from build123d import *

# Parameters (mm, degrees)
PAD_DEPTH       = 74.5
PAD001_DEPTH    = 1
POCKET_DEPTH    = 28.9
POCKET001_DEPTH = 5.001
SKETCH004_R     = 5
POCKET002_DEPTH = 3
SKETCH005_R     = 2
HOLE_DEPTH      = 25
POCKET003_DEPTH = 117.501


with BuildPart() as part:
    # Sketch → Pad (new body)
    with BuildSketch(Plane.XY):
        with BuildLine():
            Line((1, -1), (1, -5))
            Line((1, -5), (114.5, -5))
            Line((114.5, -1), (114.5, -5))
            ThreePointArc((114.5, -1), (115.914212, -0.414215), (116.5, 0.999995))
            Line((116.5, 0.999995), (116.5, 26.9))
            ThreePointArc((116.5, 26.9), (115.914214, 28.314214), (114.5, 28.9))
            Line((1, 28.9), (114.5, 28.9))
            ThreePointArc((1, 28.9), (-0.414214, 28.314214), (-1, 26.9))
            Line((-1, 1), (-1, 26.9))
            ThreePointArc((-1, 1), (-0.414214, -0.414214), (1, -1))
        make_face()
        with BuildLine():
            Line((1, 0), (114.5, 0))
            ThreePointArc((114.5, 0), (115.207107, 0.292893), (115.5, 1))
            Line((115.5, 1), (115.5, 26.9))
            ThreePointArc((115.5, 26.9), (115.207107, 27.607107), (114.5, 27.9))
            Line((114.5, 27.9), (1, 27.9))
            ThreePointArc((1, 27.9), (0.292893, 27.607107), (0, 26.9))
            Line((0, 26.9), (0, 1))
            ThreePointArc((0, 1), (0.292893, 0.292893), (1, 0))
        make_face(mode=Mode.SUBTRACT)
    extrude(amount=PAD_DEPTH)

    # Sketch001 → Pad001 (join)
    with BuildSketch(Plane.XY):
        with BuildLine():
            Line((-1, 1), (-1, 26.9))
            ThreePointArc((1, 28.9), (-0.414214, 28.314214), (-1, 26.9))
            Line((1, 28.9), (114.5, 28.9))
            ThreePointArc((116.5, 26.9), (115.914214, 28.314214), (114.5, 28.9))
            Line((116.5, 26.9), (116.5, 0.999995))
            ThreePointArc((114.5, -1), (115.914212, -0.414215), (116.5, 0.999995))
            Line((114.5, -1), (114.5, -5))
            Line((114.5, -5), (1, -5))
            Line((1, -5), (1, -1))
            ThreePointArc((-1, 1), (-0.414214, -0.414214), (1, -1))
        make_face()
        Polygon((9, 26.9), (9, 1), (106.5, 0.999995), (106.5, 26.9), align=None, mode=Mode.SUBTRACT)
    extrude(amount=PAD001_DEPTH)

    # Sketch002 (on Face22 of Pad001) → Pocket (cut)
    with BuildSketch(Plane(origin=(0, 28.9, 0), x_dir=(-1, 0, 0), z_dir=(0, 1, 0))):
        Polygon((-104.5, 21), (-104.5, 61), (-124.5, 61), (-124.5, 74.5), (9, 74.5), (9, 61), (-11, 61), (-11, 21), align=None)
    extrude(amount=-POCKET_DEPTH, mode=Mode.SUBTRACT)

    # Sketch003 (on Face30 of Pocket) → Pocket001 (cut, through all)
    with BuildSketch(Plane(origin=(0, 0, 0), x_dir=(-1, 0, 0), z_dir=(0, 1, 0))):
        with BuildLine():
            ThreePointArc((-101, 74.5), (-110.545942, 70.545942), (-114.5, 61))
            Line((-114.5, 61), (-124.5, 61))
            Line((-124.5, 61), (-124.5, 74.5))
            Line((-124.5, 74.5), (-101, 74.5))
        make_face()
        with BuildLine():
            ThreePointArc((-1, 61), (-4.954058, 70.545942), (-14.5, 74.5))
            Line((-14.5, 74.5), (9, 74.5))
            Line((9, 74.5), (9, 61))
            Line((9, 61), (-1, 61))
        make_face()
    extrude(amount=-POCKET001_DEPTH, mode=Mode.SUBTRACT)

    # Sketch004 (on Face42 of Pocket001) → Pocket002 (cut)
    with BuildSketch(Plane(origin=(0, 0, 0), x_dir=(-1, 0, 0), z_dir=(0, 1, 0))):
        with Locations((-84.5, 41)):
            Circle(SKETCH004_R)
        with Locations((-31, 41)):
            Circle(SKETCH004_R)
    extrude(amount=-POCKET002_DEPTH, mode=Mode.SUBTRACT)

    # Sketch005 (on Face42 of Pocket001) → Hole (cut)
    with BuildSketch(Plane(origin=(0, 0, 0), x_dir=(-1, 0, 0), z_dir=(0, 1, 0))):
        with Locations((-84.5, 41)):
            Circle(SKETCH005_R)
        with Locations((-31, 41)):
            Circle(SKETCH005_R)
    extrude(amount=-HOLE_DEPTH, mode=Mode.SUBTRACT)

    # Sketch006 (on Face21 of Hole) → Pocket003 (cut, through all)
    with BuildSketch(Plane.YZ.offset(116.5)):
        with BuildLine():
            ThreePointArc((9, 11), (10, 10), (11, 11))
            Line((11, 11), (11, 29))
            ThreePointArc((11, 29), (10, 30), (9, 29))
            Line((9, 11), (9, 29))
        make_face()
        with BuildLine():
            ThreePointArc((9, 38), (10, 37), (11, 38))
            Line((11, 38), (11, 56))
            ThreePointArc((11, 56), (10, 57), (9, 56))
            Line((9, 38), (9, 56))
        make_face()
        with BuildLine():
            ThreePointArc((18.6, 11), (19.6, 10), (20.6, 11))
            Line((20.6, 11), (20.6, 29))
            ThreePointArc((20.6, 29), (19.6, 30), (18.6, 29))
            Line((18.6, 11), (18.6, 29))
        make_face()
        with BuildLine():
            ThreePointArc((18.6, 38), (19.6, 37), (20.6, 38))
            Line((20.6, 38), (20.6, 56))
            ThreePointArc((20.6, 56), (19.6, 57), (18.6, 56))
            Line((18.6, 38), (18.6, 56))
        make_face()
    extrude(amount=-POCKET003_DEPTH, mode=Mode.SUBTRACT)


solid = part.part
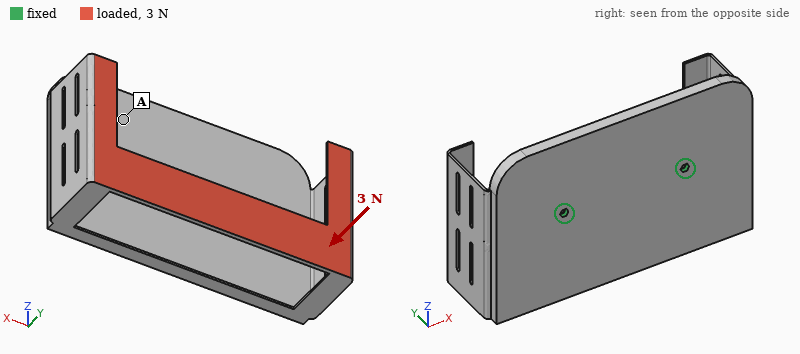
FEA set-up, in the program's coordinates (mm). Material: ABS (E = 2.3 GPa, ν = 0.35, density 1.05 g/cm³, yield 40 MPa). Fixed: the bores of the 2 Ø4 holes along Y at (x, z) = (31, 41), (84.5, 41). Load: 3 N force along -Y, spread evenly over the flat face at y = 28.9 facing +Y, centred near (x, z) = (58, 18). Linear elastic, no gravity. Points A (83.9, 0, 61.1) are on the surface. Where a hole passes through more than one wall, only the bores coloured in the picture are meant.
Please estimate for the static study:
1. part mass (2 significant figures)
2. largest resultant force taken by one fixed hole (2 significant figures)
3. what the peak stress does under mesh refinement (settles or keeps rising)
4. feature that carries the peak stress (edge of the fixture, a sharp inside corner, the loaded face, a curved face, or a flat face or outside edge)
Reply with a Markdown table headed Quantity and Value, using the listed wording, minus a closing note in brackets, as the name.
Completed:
| Quantity | Value |
|---|---|
| part mass | 51 g |
| largest resultant force taken by one fixed hole | 4.2 N |
| what the peak stress does under mesh refinement | keeps rising |
| feature that carries the peak stress | a sharp inside corner |
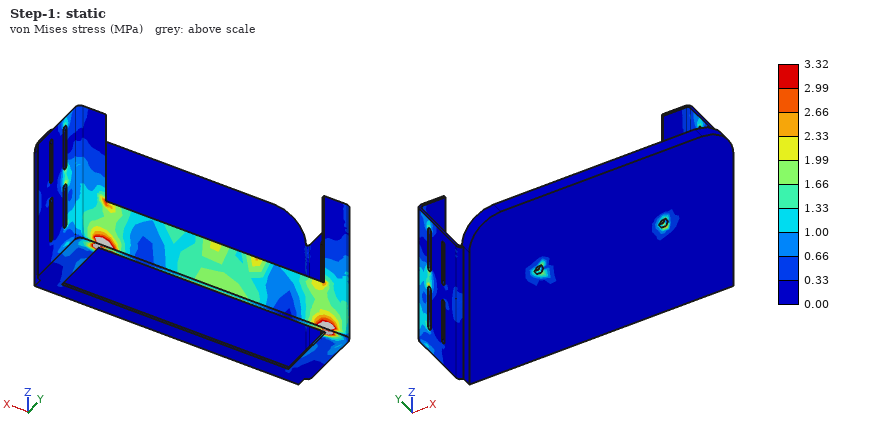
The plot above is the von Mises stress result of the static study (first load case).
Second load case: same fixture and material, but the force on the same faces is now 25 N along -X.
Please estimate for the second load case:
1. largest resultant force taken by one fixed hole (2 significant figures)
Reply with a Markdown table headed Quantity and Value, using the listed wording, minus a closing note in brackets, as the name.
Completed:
| Quantity | Value |
|---|---|
| largest resultant force taken by one fixed hole | 21 N |
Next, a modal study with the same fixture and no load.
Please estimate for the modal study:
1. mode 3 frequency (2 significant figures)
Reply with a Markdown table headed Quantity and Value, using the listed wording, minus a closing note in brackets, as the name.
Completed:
| Quantity | Value |
|---|---|
| mode 3 frequency | 300 Hz |
